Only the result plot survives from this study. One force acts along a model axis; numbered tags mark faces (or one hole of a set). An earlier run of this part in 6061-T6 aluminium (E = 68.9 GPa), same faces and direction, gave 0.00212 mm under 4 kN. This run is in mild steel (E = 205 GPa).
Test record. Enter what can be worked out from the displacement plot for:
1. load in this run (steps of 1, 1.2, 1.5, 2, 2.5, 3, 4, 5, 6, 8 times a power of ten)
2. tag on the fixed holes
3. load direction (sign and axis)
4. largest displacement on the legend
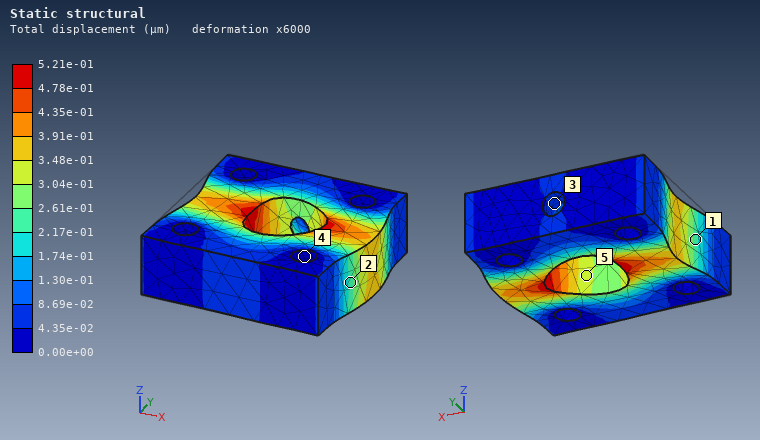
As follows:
3 kN
4
+X
5.21e-01 µm
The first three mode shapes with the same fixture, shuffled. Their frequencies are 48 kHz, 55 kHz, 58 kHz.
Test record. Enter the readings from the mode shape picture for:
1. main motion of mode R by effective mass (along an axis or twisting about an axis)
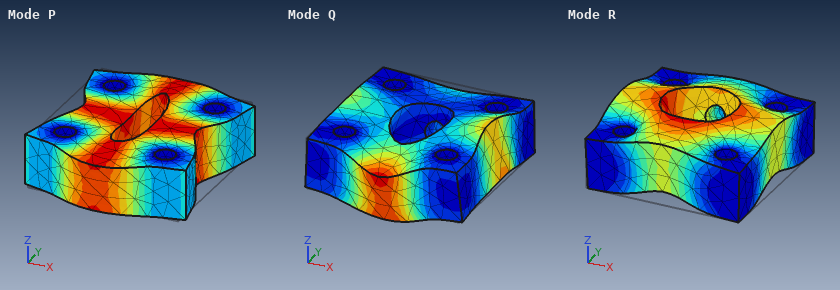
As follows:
along Z
